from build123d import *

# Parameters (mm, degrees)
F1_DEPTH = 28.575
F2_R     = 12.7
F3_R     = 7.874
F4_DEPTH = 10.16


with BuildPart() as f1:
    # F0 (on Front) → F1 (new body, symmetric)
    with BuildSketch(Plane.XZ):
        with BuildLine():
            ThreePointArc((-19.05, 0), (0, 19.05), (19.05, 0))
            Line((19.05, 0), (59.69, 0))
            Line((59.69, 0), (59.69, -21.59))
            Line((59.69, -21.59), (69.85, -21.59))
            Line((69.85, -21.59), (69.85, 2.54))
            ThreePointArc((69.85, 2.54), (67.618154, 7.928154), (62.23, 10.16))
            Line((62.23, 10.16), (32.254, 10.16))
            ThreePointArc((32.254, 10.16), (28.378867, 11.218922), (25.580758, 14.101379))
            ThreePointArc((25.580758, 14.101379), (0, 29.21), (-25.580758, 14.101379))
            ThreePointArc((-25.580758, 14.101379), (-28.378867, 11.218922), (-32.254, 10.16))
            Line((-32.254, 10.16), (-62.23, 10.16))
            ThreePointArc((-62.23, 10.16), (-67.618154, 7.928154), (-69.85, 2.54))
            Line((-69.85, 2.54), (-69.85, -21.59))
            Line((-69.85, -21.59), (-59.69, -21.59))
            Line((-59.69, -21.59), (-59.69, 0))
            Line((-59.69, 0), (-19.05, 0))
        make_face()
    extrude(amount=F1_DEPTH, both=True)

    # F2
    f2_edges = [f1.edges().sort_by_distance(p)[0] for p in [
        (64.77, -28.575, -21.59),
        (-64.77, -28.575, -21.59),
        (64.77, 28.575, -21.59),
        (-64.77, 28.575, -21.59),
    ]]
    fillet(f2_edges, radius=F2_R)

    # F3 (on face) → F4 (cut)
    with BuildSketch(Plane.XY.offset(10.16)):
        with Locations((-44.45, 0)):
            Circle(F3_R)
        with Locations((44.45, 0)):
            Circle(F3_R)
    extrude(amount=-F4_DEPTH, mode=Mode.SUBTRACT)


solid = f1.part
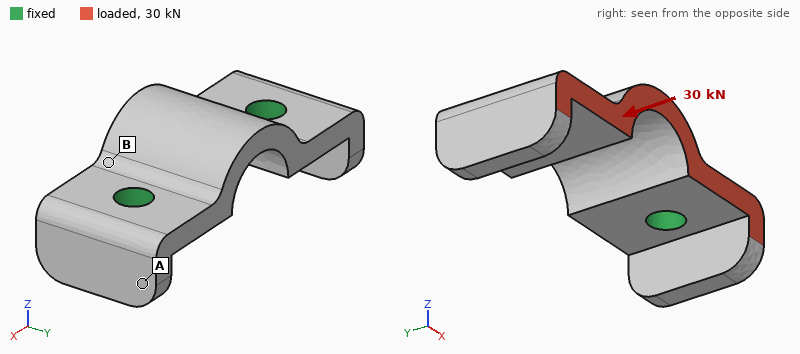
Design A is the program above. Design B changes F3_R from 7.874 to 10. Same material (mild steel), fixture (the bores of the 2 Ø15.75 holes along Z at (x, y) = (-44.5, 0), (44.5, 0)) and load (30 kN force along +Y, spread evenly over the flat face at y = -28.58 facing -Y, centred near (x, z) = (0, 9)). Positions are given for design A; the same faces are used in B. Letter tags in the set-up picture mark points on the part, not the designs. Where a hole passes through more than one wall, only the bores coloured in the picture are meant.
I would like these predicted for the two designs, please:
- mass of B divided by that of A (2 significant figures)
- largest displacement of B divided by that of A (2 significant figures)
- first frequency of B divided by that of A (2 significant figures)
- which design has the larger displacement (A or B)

0.98
0.78
1.2
A
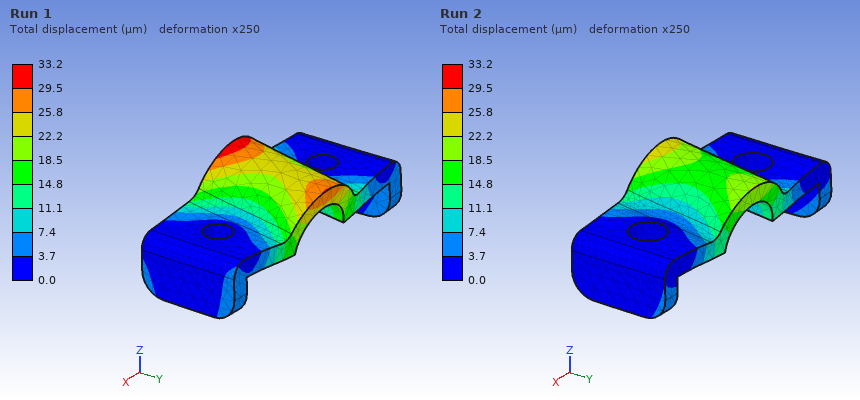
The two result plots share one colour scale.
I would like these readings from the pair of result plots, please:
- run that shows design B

Run 2
